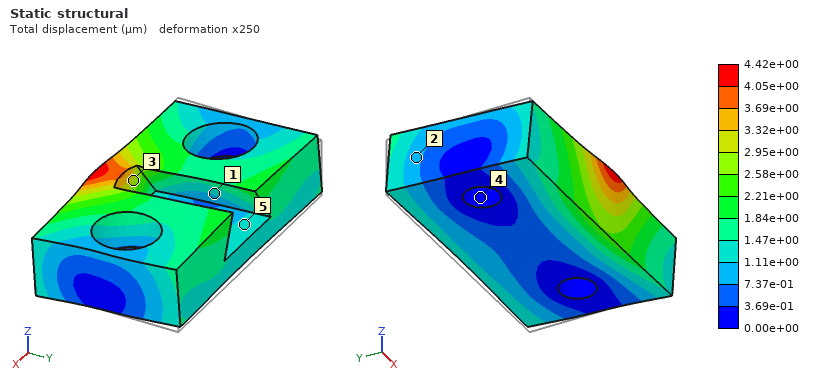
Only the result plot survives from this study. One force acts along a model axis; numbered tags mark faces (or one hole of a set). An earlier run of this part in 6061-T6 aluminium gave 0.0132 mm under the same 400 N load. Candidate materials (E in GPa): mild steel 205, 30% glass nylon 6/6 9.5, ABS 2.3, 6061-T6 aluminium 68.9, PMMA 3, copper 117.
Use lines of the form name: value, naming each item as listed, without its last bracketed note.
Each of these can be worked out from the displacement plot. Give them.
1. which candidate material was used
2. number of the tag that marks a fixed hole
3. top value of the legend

which candidate material was used: mild steel
number of the tag that marks a fixed hole: 4
top value of the legend: 4.42e+00 µm
